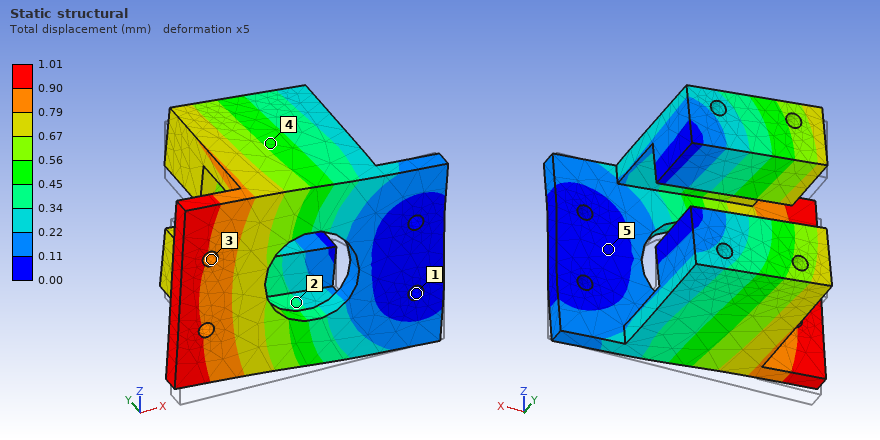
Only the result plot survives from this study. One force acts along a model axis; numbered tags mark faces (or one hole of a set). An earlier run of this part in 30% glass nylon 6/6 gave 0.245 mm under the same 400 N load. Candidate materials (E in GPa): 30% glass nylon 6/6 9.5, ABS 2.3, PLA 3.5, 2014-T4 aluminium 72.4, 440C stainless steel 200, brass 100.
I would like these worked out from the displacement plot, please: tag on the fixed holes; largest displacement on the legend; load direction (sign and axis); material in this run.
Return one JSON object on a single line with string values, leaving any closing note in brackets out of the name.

{"tag on the fixed holes": "1", "largest displacement on the legend": "1.01 mm", "load direction": "+Z", "material in this run": "ABS"}
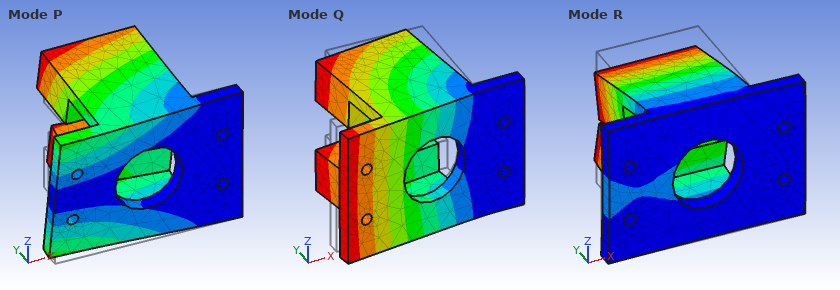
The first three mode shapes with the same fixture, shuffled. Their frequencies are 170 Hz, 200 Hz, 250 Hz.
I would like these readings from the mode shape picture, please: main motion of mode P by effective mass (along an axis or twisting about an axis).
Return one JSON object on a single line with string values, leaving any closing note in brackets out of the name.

{"main motion of mode P by effective mass": "along Z"}
